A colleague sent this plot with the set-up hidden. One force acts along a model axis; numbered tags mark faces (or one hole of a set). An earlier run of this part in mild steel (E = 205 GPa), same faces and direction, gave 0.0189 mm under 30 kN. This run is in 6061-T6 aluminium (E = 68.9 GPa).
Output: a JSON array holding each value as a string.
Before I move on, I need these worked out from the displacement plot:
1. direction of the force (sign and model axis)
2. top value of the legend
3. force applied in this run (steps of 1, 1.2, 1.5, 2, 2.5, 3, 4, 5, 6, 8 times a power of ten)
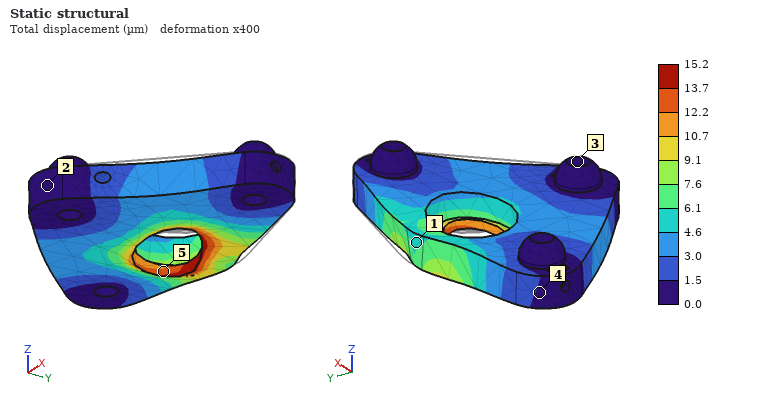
["-X", "15.2 µm", "8 kN"]
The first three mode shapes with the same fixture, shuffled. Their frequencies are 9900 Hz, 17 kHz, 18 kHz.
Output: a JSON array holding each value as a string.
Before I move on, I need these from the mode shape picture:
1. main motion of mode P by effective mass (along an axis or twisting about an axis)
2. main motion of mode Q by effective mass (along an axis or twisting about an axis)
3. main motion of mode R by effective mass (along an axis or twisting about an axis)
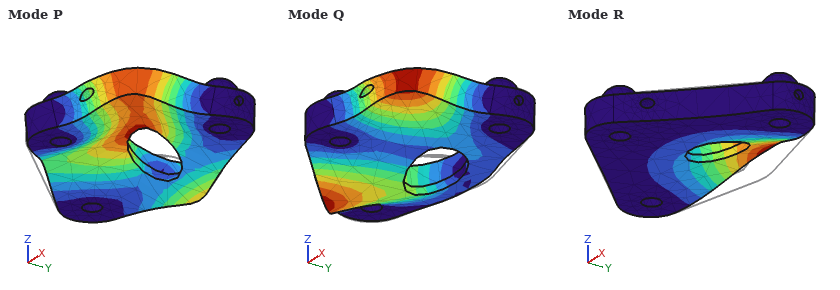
["along Z", "twisting about Y", "along Z"]
